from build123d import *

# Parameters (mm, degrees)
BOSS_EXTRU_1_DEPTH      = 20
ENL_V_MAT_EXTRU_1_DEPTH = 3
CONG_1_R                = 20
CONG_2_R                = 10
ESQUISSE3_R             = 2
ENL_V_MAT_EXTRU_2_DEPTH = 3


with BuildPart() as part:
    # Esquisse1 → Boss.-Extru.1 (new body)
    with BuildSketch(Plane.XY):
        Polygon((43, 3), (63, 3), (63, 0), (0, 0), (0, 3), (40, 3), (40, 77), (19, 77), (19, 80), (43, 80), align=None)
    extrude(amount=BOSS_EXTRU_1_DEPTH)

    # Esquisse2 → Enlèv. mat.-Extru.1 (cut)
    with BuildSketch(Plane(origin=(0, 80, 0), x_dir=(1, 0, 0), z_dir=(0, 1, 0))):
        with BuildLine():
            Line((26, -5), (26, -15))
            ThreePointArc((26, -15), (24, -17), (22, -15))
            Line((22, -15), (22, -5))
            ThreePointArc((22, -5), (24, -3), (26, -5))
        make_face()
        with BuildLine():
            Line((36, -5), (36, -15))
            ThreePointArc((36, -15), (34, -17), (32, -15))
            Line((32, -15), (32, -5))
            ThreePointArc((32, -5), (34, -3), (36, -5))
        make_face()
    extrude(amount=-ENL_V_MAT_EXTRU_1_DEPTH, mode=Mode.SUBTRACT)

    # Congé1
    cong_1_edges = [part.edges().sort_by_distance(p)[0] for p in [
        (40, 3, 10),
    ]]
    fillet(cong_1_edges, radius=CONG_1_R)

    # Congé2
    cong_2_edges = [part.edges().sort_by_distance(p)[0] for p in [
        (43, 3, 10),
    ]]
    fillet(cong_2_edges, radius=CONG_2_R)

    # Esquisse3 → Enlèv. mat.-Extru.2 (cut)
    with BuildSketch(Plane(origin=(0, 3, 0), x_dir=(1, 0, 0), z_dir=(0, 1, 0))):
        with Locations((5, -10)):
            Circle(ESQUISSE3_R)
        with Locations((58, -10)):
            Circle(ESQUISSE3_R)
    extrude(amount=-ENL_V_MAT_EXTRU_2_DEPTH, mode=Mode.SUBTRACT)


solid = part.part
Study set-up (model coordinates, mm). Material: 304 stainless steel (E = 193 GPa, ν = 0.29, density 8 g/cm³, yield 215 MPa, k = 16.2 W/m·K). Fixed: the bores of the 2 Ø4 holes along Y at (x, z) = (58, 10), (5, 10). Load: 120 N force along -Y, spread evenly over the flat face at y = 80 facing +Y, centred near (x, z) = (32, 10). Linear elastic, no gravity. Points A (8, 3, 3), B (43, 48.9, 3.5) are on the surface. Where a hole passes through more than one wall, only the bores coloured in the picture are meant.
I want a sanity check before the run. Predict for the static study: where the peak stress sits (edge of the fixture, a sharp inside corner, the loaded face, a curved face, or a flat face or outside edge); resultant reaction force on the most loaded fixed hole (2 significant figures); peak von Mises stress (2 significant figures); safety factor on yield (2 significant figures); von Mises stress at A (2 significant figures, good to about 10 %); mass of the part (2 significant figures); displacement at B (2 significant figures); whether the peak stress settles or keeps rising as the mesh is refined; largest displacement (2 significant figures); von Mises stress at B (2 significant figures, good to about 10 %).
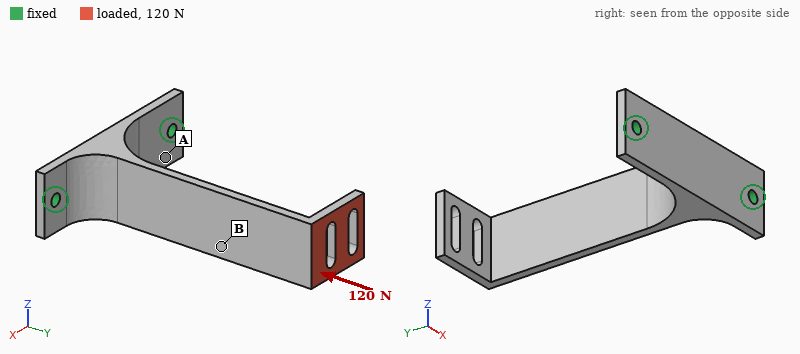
a curved face
92 N
92 MPa
2.3
8.3 MPa
91 g
0.079 mm
settles
0.37 mm
38 MPa
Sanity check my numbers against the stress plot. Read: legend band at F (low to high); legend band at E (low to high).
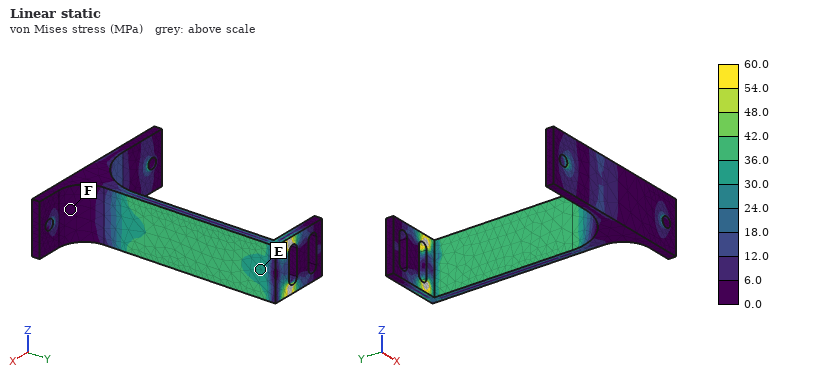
0.0 to 6.0 MPa
30.0 to 36.0 MPa
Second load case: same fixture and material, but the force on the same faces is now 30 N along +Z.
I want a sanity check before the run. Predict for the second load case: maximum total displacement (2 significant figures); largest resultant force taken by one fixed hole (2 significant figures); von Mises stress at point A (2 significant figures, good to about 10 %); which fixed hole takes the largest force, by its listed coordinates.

0.12 mm
20 N
12 MPa
(58, 10)
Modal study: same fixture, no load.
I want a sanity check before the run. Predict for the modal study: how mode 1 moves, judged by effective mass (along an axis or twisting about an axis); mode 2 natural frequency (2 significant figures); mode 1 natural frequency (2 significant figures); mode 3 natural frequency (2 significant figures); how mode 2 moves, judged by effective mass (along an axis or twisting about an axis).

along X
650 Hz
400 Hz
1800 Hz
along Z
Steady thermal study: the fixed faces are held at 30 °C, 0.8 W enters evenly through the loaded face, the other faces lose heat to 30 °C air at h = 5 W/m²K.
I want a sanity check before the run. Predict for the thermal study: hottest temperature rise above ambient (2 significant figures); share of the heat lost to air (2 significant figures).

49 K
58 %
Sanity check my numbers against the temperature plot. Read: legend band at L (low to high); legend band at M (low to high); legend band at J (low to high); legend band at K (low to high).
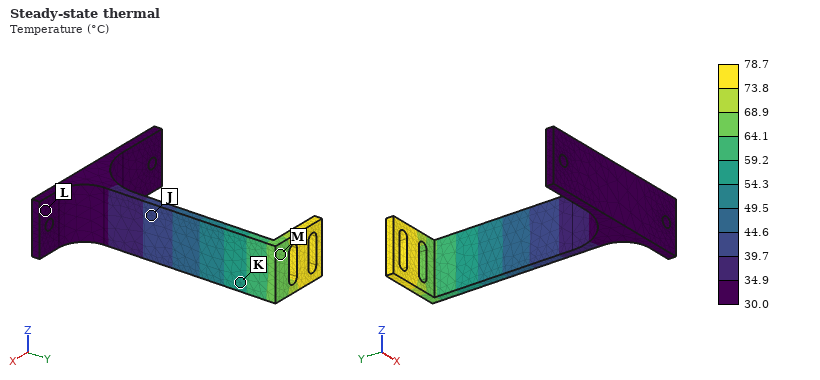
30.0 to 34.9 °C
64.1 to 68.9 °C
39.7 to 44.6 °C
54.3 to 59.2 °C
